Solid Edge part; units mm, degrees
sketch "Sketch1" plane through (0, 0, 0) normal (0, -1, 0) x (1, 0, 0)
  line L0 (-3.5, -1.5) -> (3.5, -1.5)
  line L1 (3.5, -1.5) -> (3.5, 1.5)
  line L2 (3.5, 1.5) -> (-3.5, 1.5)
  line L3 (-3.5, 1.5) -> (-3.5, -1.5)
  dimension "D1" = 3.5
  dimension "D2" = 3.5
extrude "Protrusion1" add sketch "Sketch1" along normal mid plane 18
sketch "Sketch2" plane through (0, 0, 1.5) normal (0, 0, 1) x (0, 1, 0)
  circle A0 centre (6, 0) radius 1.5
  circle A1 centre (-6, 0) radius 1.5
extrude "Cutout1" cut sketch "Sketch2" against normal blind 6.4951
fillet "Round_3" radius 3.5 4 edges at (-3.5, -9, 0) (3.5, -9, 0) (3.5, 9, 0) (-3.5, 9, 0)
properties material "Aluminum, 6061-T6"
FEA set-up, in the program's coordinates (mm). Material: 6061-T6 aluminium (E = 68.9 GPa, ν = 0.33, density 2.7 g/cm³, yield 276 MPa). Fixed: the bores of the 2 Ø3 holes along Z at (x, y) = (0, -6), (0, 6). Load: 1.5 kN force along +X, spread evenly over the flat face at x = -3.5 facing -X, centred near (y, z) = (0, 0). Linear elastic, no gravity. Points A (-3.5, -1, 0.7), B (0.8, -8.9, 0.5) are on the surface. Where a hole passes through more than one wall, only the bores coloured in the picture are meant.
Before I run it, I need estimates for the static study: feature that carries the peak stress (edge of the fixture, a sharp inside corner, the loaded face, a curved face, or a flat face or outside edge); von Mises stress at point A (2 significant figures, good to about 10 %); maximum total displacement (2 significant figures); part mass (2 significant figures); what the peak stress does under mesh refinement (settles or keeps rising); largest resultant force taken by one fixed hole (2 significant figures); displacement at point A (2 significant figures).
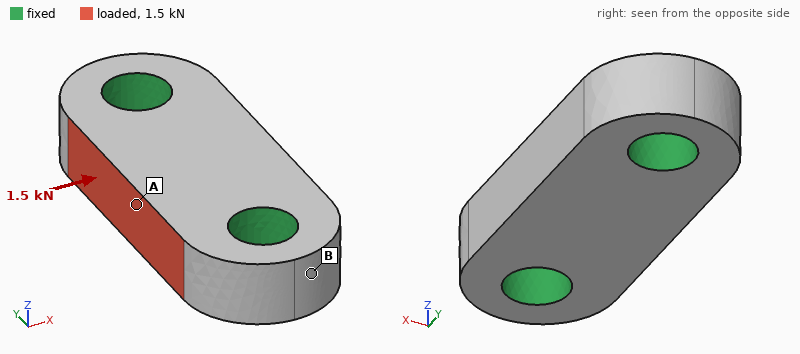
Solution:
edge of the fixture
57 MPa
6.5 µm
0.82 g
keeps rising
770 N
6.2 µm
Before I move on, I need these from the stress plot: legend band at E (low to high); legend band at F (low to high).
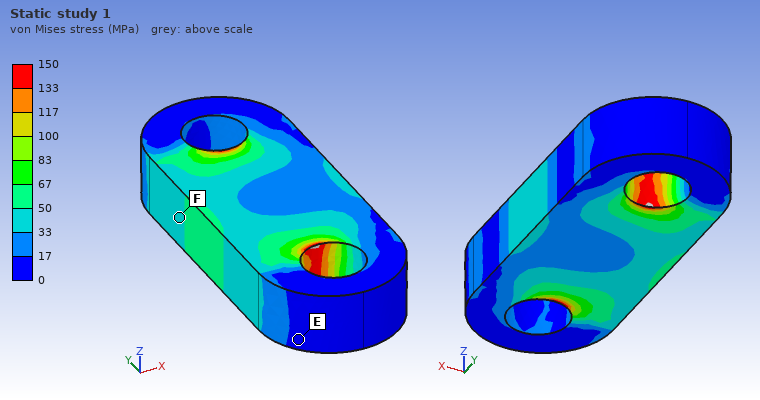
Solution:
0 to 17 MPa
33 to 50 MPa
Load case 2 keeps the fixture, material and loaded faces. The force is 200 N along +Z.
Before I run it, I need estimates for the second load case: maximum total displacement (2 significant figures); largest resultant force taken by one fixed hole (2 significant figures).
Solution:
4.4 µm
100 N
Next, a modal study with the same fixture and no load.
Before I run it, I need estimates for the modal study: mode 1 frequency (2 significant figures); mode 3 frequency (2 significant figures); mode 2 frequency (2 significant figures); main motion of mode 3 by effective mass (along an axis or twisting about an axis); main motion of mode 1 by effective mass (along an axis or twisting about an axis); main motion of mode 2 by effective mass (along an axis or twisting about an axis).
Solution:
98 kHz
120 kHz
110 kHz
along X
along Z
twisting about Y
